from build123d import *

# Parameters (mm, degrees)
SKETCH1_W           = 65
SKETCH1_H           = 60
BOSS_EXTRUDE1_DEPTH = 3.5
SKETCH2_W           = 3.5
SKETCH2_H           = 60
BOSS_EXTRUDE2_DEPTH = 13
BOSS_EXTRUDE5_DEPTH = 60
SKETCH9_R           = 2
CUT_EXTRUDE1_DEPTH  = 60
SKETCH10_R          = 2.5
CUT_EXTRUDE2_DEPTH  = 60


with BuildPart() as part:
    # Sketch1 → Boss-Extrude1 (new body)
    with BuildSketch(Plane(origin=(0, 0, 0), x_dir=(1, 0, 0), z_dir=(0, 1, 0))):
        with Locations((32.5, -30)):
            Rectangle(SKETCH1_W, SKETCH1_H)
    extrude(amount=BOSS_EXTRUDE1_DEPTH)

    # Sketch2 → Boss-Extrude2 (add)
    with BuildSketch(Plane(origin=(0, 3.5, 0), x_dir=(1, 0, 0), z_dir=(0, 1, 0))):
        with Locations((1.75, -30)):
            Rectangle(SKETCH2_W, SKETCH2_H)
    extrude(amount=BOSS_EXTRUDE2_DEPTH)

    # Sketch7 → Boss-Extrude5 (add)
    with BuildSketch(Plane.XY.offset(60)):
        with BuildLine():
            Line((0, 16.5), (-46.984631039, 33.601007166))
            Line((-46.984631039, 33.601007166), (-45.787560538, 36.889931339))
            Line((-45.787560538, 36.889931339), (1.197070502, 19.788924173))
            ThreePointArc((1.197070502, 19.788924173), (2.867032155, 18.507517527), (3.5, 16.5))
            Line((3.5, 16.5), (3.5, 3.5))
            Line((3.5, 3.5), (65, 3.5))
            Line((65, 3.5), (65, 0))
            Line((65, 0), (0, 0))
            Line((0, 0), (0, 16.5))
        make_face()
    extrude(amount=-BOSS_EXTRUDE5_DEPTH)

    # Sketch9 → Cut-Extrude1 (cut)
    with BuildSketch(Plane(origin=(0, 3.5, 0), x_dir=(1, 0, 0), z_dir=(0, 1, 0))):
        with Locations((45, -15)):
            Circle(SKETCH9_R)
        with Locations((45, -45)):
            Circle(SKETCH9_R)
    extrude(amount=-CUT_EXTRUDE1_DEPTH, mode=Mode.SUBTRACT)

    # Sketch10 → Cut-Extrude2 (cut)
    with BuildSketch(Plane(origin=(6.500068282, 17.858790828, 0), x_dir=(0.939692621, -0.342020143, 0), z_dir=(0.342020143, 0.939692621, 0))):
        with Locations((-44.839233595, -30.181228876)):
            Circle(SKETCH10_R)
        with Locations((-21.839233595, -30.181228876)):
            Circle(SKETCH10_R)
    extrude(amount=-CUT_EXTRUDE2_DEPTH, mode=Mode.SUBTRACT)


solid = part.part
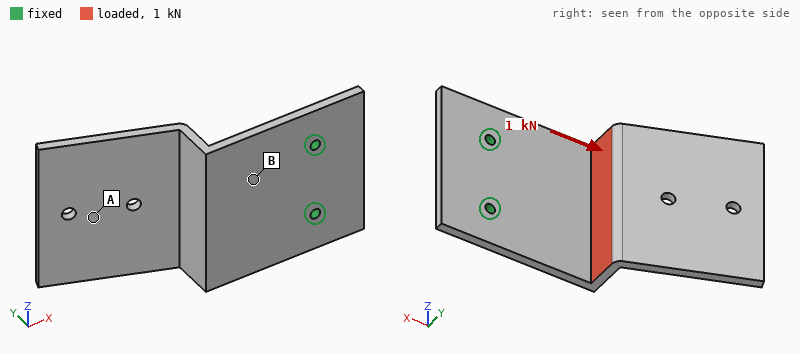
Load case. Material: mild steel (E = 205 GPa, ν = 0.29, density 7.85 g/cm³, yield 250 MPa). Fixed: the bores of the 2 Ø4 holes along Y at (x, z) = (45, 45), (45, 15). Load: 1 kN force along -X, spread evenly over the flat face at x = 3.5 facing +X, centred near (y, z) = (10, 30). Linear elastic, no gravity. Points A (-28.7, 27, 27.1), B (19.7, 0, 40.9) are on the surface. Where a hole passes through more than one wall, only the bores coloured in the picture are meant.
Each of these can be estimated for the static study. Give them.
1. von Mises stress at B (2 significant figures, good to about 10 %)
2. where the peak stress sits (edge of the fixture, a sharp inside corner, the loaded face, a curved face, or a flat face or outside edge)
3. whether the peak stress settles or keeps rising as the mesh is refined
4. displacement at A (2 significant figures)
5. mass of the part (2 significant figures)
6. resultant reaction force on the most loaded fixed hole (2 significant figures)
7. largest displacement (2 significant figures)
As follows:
55 MPa
edge of the fixture
keeps rising
0.49 mm
210 g
500 N
0.66 mm
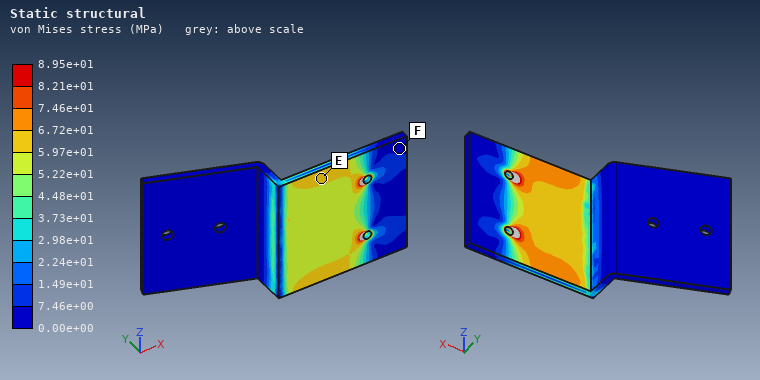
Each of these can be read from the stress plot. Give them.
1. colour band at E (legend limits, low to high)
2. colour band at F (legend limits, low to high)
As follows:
5.97e+01 to 6.72e+01 MPa
0.00e+00 to 7.46e+00 MPa
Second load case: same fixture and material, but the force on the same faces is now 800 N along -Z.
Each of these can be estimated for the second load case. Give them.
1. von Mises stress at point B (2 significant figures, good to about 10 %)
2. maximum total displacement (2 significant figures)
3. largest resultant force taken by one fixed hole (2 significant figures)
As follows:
26 MPa
0.12 mm
1.1 kN
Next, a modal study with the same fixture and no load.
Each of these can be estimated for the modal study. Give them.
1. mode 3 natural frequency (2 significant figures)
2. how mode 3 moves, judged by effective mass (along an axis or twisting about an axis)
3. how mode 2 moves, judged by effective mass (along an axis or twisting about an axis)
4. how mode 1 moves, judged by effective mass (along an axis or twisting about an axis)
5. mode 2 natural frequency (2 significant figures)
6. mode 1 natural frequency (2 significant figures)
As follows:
1400 Hz
along Y
along Z
along Y
860 Hz
280 Hz
